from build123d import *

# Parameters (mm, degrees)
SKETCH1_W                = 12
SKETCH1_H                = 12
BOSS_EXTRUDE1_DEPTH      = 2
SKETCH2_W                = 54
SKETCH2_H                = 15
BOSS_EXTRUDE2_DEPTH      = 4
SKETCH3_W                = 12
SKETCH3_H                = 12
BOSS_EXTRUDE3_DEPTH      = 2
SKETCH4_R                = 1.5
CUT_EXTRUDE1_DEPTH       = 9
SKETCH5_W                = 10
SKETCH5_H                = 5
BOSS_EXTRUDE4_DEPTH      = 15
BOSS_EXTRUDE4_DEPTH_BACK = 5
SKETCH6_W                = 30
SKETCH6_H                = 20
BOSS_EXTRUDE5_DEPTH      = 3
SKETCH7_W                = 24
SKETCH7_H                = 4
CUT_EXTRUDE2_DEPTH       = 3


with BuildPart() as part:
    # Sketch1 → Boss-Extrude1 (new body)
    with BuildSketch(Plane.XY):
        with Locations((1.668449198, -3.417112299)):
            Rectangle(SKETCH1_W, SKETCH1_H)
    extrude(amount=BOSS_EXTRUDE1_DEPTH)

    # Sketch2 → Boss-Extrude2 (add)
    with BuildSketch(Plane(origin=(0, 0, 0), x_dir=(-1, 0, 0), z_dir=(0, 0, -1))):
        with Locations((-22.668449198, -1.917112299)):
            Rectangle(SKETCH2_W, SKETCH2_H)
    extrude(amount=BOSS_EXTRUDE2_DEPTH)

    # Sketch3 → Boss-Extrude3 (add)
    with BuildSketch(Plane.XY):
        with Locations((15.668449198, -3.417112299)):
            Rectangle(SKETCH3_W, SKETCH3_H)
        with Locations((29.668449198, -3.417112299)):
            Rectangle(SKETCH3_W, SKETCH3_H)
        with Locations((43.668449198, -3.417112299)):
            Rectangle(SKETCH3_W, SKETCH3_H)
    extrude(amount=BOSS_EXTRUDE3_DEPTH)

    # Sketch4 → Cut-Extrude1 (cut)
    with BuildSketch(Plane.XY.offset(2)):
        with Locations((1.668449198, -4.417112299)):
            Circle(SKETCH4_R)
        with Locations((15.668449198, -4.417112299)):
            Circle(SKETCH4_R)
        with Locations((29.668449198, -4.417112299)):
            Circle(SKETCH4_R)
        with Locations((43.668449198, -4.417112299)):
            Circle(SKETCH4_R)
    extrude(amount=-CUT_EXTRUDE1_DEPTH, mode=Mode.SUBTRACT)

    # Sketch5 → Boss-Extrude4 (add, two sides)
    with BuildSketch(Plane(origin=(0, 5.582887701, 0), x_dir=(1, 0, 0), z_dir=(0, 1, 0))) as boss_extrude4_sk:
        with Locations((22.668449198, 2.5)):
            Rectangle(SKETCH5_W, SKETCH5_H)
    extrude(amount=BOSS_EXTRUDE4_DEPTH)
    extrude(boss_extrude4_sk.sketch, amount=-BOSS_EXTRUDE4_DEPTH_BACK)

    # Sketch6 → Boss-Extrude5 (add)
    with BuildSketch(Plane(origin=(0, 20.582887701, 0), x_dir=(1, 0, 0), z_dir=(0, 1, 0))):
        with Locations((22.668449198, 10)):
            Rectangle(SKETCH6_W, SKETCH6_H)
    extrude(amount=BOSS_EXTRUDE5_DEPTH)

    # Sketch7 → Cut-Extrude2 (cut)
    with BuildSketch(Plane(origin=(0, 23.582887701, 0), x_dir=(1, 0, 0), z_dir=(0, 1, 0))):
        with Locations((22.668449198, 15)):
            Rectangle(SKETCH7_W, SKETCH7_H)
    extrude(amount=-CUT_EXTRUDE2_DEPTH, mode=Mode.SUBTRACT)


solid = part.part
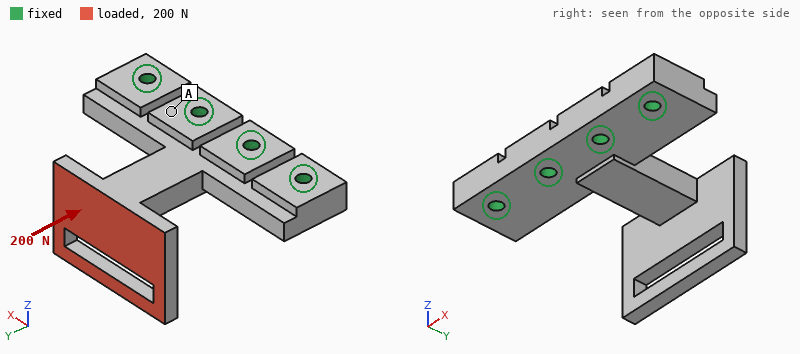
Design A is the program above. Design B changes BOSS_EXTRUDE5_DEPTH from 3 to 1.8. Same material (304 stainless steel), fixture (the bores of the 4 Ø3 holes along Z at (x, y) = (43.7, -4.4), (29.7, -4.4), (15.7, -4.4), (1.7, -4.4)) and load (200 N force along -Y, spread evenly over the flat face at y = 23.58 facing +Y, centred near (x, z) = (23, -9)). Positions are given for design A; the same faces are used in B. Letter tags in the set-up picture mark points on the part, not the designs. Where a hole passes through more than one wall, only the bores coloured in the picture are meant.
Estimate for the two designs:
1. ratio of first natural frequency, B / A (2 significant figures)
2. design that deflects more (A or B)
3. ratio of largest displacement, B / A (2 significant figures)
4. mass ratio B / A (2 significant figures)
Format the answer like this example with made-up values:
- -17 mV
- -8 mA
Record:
- 1.2
- B
- 1.9
- 0.91
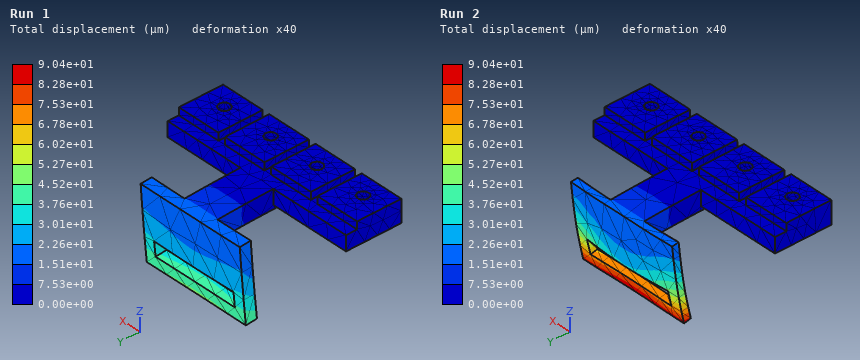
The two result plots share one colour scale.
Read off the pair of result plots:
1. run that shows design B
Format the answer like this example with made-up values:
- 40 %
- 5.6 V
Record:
- Run 2
